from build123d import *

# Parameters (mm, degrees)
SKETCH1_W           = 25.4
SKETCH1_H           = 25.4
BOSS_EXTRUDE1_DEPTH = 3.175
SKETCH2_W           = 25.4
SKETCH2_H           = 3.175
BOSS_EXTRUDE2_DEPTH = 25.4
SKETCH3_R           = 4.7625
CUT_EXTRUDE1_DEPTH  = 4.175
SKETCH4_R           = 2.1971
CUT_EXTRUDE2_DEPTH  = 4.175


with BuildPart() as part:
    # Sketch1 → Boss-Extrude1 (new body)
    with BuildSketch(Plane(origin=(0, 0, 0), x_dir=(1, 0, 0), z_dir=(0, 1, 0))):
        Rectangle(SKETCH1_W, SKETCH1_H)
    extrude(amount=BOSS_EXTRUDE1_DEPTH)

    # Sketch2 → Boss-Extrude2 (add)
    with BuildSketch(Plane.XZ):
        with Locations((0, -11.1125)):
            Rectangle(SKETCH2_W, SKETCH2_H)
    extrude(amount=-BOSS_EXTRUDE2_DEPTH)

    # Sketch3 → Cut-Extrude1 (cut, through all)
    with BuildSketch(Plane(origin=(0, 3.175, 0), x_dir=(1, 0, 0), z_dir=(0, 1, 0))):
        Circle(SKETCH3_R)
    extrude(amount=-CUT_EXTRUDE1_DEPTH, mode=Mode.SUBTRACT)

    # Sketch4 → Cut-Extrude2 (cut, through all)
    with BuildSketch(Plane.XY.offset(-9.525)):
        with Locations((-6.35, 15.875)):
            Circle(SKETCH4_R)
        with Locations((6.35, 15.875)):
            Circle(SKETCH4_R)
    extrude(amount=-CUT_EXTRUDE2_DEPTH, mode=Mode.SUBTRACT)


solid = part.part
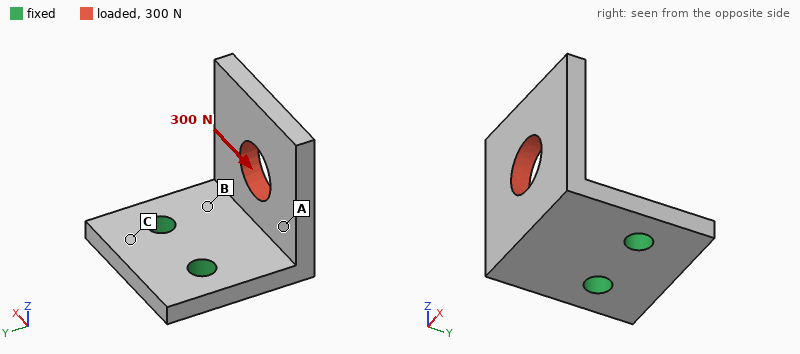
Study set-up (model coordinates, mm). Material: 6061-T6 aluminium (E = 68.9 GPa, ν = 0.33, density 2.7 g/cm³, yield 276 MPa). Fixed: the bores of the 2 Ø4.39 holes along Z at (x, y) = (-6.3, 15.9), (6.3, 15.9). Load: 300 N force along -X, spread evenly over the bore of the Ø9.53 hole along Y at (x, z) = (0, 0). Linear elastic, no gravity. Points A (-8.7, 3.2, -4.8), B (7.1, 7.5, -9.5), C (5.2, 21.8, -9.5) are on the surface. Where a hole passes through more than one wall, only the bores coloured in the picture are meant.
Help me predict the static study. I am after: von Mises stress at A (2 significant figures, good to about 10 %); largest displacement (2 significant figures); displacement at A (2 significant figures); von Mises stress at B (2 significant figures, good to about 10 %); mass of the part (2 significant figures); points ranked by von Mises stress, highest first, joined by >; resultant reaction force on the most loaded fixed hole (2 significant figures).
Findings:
22 MPa
88 µm
34 µm
41 MPa
9.5 g
B > A > C
350 N
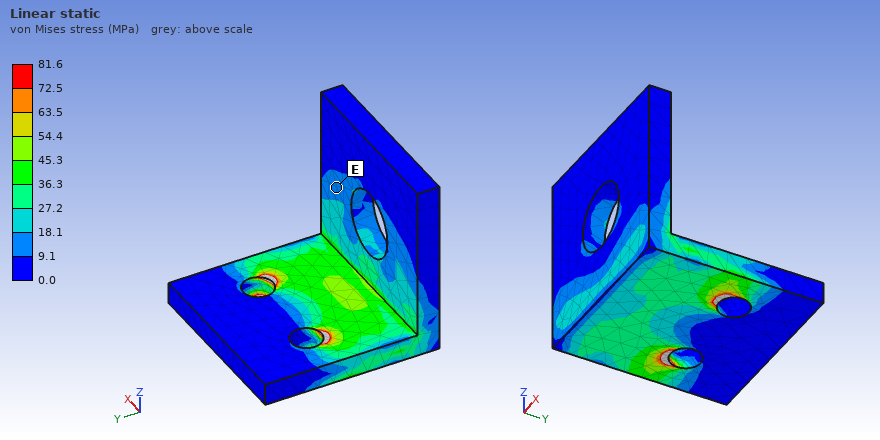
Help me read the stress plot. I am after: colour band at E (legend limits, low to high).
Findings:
9.1 to 18.1 MPa
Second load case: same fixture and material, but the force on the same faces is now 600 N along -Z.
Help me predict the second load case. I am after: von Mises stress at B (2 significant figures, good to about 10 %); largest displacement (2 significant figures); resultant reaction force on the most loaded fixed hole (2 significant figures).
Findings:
75 MPa
0.28 mm
300 N
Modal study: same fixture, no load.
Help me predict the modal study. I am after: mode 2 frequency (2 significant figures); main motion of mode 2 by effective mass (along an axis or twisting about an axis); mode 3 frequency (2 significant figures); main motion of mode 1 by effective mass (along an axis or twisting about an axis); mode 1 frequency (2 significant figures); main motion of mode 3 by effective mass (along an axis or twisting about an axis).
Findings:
4600 Hz
along X
7800 Hz
along Y
2500 Hz
along Z
